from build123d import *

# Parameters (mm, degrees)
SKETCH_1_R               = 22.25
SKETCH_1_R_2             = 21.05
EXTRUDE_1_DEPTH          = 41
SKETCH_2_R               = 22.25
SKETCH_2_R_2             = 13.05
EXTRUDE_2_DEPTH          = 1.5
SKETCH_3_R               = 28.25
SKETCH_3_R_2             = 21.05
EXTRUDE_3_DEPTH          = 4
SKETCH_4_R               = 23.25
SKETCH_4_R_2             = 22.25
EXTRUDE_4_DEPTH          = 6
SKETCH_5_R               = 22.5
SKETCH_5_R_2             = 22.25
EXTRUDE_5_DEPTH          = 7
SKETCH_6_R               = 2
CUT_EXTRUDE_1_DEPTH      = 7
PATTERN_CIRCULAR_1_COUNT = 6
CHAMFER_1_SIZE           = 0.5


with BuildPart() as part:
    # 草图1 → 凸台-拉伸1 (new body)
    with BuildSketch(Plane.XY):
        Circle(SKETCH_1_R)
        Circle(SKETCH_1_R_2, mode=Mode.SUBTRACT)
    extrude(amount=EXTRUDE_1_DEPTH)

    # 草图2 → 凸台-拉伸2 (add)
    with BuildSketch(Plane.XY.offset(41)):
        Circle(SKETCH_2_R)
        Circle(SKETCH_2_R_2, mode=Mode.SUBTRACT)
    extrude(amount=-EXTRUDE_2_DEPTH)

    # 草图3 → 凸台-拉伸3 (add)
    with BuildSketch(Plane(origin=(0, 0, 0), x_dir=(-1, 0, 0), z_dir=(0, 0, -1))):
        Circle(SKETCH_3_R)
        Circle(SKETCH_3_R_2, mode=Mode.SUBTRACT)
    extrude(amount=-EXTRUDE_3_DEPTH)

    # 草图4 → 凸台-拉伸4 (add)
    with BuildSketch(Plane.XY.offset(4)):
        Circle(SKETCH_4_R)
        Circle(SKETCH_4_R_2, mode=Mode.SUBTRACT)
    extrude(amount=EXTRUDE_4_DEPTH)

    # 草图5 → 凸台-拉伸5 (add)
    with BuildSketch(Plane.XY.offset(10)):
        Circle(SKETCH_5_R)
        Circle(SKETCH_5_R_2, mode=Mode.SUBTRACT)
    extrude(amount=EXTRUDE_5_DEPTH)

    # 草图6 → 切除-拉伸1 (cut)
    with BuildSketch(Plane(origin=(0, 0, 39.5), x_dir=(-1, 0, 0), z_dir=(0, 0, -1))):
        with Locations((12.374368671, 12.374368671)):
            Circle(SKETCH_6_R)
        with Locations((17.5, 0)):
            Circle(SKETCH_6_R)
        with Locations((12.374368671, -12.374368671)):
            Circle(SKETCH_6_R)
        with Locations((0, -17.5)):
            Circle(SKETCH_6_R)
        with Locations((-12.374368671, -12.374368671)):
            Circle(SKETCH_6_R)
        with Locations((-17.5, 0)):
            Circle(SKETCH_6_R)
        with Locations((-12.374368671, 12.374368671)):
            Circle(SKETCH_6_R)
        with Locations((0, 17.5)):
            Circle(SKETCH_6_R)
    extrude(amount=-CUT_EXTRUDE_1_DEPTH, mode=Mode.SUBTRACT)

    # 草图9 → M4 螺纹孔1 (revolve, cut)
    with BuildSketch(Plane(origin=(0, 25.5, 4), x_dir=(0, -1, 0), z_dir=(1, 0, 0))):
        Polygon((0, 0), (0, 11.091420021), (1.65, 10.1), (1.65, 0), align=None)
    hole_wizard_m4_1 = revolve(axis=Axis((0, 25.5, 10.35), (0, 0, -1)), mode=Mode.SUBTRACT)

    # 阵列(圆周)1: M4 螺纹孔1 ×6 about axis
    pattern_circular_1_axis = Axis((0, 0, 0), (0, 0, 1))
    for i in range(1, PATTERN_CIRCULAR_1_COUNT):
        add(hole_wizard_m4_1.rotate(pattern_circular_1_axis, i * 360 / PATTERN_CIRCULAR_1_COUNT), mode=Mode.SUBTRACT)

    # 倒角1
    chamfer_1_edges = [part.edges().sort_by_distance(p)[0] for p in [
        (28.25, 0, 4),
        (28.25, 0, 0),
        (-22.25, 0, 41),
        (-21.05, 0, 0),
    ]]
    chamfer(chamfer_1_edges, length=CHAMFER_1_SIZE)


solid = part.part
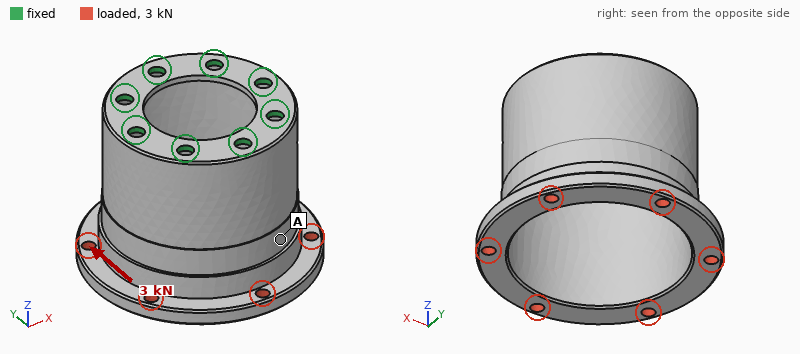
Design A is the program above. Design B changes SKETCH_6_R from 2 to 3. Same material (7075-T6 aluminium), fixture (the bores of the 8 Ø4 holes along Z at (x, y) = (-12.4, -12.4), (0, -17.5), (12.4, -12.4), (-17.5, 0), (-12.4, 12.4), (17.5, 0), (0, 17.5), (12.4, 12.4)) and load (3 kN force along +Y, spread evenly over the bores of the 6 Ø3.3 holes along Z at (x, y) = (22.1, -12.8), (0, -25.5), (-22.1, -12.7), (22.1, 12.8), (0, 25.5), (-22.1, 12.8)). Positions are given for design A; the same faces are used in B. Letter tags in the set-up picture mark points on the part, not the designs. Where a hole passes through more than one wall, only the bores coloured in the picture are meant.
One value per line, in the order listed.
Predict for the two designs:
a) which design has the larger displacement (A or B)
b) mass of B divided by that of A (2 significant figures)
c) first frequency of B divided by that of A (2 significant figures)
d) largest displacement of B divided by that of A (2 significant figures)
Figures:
A
0.98
1.3
0.66
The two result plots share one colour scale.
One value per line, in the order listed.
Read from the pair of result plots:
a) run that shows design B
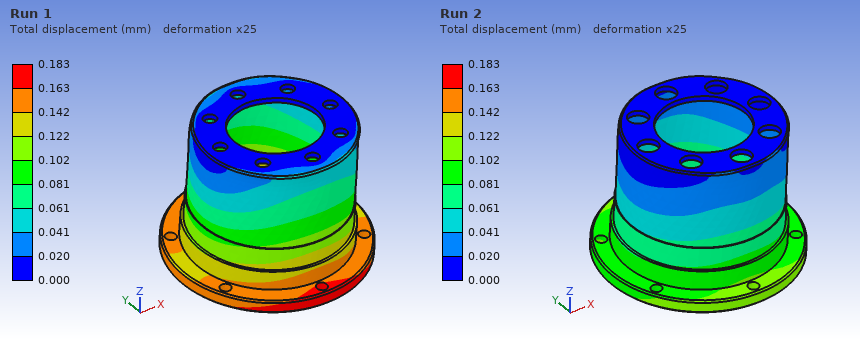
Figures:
Run 2
